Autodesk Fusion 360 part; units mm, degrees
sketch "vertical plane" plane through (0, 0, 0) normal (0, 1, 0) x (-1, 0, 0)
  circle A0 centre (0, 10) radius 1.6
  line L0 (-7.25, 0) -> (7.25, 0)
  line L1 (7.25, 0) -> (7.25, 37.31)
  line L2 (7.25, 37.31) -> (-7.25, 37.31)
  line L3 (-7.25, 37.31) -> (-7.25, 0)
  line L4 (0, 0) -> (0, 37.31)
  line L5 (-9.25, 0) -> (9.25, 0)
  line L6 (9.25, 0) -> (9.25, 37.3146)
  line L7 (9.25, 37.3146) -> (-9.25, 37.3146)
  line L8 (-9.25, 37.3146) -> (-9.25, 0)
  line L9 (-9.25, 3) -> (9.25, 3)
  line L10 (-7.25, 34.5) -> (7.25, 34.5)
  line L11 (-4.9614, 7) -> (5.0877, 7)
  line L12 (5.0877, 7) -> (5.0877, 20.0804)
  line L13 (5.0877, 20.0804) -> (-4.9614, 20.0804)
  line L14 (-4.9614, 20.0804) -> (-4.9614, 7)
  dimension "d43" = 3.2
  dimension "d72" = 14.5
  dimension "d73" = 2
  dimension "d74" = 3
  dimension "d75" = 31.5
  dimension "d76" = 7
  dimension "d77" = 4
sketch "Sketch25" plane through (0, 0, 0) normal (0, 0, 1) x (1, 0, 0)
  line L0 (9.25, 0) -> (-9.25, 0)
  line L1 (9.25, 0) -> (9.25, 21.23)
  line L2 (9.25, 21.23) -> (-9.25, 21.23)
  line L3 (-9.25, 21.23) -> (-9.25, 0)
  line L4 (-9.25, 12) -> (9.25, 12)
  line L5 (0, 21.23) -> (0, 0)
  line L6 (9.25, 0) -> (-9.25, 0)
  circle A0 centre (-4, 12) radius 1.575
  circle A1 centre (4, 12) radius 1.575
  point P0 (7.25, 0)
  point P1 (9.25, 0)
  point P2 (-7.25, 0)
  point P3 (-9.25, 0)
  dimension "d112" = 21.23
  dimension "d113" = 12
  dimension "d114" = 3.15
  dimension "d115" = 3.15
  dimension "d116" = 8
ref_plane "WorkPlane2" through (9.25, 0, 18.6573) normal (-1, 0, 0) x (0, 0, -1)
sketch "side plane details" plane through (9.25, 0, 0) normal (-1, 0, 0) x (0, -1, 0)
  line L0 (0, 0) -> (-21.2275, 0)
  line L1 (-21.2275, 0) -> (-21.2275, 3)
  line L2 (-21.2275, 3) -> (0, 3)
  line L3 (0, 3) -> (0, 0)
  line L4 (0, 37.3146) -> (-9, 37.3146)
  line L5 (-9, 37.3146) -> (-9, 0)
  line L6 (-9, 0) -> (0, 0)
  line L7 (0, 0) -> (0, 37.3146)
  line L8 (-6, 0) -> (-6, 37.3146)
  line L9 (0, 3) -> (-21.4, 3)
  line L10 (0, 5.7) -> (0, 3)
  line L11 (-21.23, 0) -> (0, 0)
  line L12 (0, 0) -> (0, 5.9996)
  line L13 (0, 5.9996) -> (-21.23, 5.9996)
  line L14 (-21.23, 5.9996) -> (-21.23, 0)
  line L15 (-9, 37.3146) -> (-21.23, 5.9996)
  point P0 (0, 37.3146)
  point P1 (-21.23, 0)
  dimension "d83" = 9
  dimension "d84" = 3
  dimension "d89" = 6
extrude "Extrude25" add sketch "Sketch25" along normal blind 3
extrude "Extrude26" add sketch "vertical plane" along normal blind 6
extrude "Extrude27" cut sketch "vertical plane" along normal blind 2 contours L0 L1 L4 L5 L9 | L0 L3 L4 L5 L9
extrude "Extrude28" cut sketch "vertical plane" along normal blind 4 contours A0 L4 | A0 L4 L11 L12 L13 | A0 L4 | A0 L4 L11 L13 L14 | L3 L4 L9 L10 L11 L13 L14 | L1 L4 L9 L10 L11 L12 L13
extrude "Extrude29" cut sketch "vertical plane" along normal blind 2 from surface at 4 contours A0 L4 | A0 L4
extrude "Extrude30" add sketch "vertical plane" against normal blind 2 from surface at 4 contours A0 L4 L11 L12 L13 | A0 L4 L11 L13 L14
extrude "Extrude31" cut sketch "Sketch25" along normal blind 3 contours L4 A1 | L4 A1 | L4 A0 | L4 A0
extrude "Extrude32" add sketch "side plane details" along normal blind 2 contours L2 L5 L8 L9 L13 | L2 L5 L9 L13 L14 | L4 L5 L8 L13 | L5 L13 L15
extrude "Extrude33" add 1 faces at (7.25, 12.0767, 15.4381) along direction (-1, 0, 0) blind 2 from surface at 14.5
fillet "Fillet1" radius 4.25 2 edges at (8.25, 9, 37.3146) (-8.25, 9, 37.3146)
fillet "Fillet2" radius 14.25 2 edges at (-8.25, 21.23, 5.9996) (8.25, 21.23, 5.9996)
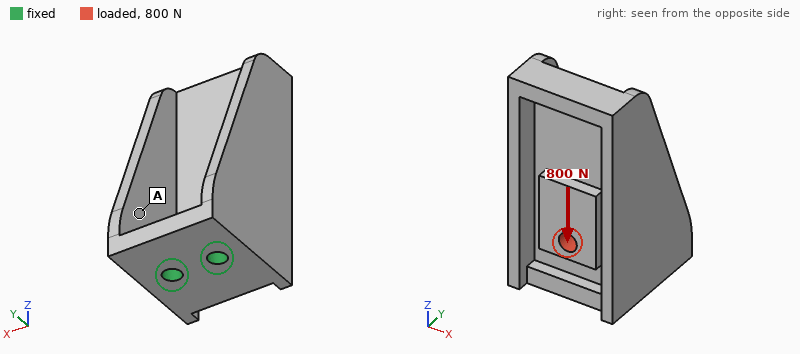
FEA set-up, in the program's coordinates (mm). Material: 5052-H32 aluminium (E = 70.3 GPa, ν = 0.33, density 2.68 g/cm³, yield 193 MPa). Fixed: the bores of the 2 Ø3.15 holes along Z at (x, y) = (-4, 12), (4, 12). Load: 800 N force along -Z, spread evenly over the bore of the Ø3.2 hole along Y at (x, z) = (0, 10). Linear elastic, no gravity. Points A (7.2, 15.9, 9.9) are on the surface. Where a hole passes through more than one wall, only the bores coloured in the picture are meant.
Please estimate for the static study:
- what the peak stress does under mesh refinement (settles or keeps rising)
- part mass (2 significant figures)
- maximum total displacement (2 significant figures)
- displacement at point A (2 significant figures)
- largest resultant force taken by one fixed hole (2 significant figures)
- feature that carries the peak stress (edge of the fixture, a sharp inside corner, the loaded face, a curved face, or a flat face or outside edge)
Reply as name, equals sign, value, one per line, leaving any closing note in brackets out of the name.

what the peak stress does under mesh refinement = keeps rising
part mass = 12 g
maximum total displacement = 96 µm
displacement at point A = 22 µm
largest resultant force taken by one fixed hole = 400 N
feature that carries the peak stress = edge of the fixture
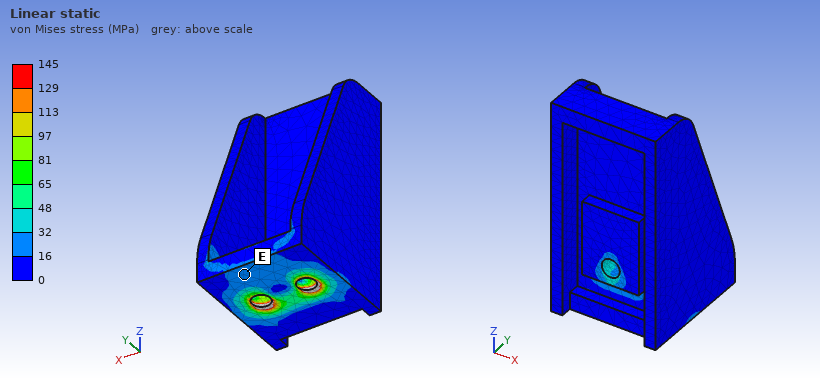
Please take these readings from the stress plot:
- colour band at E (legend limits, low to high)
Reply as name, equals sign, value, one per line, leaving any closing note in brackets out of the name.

colour band at E = 16 to 32 MPa
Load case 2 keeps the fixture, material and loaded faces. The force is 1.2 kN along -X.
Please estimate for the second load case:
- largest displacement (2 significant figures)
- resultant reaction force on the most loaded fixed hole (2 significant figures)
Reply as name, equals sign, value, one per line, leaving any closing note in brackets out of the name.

largest displacement = 0.13 mm
resultant reaction force on the most loaded fixed hole = 1.3 kN
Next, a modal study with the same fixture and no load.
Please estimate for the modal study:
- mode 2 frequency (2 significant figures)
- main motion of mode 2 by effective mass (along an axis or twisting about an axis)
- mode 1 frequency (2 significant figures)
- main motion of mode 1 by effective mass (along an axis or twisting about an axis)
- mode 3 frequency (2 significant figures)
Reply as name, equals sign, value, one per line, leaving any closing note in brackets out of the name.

mode 2 frequency = 3900 Hz
main motion of mode 2 by effective mass = along X
mode 1 frequency = 3500 Hz
main motion of mode 1 by effective mass = along Y
mode 3 frequency = 9000 Hz
